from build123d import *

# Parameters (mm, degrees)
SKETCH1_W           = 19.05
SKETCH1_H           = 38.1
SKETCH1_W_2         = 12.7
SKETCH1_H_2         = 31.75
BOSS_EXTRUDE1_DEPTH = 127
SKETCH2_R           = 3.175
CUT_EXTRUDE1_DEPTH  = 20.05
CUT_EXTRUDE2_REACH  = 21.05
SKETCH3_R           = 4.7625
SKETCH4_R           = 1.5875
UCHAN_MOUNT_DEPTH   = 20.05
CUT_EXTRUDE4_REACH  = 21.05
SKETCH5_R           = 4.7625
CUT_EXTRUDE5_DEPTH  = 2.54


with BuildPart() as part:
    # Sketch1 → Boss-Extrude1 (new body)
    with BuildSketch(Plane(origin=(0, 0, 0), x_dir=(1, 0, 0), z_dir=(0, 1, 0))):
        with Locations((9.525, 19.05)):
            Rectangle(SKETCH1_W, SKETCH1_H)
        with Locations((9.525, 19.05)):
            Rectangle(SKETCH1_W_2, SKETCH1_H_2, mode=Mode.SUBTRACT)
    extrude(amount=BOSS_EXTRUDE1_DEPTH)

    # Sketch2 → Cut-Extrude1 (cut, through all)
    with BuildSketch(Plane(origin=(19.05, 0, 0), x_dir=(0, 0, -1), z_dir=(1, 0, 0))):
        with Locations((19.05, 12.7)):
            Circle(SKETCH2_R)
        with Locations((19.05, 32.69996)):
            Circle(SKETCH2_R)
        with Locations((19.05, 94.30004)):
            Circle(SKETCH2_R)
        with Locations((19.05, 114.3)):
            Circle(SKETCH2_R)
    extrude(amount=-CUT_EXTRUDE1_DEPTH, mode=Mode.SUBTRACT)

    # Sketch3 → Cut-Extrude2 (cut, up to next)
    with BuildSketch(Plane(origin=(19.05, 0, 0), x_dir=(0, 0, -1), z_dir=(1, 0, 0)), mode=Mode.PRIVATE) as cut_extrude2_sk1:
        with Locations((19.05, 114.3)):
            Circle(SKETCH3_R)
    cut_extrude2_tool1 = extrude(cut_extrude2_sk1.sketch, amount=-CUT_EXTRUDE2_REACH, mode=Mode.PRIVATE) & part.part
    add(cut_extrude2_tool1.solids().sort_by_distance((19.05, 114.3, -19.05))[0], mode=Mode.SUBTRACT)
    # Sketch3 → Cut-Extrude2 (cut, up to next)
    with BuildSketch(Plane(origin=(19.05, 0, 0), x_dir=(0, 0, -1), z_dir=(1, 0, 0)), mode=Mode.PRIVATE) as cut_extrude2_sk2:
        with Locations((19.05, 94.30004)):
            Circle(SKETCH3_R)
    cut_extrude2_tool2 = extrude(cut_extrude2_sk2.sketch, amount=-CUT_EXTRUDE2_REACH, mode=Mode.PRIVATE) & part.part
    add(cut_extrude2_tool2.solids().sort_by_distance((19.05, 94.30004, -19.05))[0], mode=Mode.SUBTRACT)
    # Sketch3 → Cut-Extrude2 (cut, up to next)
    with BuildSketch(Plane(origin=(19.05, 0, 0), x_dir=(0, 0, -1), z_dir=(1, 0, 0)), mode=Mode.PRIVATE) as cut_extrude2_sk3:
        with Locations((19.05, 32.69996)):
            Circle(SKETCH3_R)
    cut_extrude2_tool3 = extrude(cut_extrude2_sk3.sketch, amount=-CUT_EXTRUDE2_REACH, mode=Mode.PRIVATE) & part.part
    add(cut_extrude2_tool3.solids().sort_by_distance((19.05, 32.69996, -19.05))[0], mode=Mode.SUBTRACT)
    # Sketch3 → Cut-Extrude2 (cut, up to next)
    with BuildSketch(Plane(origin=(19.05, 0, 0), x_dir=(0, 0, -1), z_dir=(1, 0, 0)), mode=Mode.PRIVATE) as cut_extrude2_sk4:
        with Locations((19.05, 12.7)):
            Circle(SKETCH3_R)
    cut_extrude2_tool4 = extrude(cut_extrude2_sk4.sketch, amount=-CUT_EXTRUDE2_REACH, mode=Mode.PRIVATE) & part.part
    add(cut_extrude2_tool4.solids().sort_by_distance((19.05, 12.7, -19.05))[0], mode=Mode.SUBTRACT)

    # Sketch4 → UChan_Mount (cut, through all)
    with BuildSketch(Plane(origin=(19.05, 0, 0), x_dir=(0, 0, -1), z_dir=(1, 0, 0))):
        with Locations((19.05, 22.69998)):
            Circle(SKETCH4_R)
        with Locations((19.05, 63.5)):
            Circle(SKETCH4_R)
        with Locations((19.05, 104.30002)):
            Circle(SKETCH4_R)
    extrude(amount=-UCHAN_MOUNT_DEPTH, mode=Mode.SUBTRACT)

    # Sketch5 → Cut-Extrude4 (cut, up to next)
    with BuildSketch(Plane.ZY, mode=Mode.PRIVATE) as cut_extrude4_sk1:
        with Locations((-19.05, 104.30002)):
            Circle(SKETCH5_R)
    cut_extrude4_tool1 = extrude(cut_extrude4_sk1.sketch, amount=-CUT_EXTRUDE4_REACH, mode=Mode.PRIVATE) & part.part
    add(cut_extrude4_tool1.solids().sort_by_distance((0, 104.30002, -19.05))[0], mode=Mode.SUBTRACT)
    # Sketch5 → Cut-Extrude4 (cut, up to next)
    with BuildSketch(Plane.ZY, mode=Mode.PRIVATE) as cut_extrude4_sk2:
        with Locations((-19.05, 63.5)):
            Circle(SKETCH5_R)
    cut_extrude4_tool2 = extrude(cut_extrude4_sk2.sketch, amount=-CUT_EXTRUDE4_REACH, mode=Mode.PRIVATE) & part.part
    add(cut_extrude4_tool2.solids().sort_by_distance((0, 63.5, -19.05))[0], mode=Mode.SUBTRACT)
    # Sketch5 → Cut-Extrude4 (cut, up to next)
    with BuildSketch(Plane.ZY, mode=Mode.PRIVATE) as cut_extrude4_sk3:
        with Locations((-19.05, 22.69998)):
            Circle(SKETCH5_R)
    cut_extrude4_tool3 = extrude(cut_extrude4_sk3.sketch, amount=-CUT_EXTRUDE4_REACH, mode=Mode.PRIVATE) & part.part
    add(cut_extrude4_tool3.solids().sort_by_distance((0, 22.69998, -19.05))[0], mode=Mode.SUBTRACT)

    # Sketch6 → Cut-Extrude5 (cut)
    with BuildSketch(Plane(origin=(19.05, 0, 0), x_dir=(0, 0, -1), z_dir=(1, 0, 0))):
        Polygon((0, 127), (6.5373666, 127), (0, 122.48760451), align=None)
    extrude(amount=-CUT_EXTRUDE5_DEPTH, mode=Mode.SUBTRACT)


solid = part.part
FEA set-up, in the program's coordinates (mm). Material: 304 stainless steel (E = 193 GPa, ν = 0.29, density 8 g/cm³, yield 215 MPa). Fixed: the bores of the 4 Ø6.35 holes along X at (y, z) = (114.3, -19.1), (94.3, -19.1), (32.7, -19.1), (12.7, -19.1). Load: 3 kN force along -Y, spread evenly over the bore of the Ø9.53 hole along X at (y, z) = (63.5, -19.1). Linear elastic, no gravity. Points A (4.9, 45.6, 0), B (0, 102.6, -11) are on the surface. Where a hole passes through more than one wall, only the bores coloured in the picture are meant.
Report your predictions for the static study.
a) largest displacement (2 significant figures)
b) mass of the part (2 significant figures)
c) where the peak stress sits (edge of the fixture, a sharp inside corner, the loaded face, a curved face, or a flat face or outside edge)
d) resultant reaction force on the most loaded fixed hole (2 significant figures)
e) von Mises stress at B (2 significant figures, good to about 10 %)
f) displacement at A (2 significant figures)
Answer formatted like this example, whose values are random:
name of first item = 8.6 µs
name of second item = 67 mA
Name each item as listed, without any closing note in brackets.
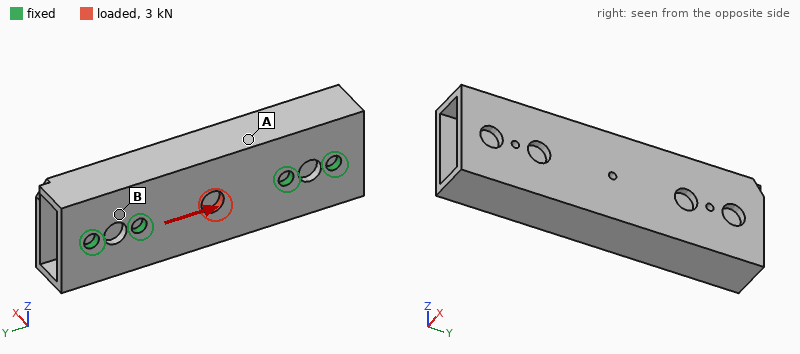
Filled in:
largest displacement = 3.3 µm
mass of the part = 310 g
where the peak stress sits = the loaded face
resultant reaction force on the most loaded fixed hole = 1.2 kN
von Mises stress at B = 7.6 MPa
displacement at A = 1.3 µm
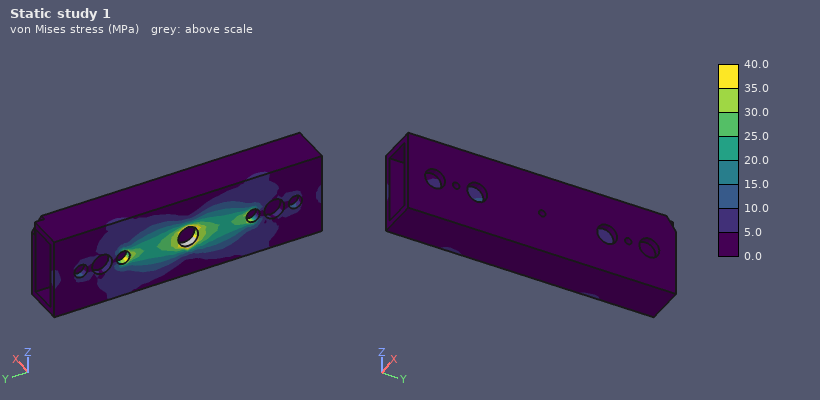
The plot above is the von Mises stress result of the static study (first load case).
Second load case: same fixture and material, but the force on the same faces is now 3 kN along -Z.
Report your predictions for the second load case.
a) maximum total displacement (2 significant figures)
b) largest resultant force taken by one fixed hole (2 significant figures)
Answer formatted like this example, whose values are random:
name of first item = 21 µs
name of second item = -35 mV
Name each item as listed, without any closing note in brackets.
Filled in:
maximum total displacement = 7.6 µm
largest resultant force taken by one fixed hole = 1.7 kN
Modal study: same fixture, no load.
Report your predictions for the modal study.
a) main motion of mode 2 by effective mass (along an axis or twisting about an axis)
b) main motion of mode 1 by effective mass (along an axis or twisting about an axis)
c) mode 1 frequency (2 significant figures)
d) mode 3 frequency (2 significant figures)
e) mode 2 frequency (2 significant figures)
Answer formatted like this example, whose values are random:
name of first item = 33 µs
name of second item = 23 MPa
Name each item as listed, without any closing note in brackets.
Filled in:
main motion of mode 2 by effective mass = along X
main motion of mode 1 by effective mass = along Z
mode 1 frequency = 2100 Hz
mode 3 frequency = 4400 Hz
mode 2 frequency = 3900 Hz
